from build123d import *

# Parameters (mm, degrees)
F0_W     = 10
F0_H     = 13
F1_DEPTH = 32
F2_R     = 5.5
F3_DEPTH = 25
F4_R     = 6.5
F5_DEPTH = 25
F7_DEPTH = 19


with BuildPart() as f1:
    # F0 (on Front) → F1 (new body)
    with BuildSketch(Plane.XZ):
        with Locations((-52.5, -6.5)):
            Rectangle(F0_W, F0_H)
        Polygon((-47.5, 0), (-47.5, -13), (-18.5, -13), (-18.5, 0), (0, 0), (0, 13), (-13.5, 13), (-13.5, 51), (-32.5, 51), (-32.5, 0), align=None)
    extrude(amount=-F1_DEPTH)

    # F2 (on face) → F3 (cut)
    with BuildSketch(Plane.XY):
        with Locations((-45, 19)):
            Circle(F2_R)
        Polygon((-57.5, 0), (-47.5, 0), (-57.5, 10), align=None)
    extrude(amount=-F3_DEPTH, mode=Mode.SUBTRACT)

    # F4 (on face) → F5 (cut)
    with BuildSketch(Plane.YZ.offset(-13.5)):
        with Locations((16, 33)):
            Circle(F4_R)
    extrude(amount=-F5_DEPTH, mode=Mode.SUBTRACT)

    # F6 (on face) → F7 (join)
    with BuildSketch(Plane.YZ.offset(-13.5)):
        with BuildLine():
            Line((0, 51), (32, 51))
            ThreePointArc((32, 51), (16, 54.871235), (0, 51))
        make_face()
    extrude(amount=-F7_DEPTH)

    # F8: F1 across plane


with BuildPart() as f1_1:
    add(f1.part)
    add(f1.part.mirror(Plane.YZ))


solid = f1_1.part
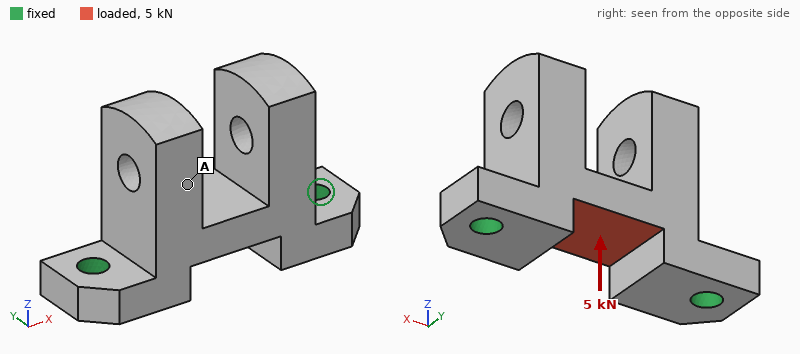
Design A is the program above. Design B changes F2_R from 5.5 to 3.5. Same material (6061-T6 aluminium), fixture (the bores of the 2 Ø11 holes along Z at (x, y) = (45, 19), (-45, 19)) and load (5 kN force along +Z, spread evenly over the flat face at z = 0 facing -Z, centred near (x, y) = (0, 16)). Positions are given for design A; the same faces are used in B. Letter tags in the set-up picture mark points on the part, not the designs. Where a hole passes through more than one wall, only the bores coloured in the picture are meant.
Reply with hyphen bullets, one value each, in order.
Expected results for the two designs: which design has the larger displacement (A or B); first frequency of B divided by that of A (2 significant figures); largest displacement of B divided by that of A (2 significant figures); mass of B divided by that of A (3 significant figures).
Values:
- B
- 0.87
- 1.2
- 1.01
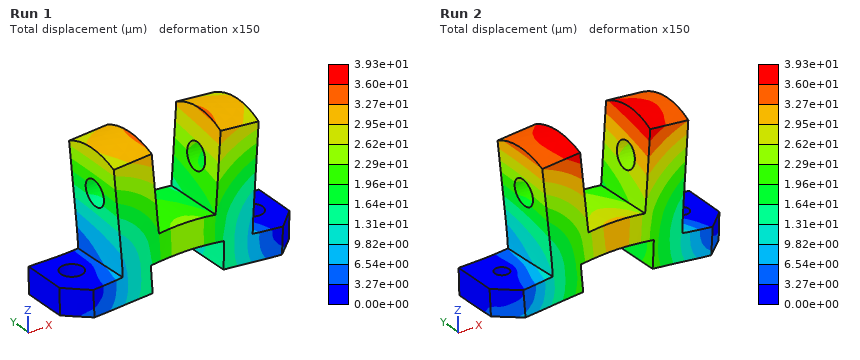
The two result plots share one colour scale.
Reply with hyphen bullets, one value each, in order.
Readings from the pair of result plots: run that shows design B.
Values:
- Run 2
